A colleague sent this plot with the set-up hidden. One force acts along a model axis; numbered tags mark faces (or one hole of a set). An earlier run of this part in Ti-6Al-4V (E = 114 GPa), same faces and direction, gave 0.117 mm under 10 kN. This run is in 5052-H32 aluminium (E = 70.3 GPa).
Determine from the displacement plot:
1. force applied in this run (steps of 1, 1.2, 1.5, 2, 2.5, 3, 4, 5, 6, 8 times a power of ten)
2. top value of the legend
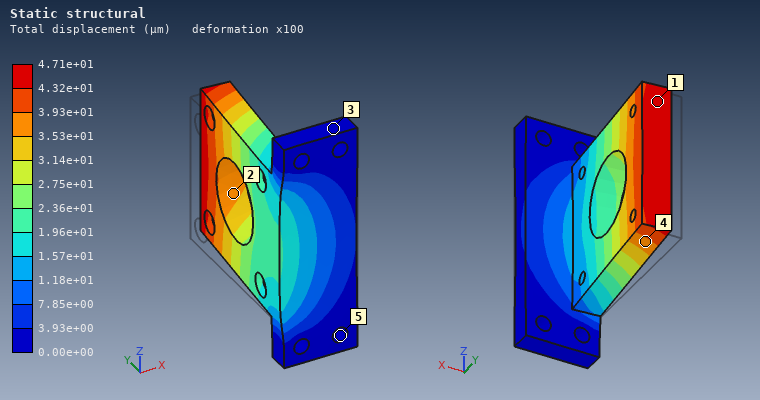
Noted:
2.5 kN
4.71e+01 µm
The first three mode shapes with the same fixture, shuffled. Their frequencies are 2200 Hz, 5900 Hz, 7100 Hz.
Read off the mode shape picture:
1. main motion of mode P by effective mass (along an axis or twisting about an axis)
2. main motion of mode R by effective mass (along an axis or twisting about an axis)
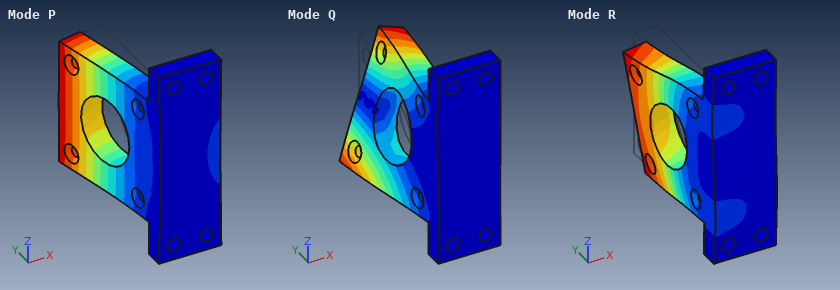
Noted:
along X
along Z
